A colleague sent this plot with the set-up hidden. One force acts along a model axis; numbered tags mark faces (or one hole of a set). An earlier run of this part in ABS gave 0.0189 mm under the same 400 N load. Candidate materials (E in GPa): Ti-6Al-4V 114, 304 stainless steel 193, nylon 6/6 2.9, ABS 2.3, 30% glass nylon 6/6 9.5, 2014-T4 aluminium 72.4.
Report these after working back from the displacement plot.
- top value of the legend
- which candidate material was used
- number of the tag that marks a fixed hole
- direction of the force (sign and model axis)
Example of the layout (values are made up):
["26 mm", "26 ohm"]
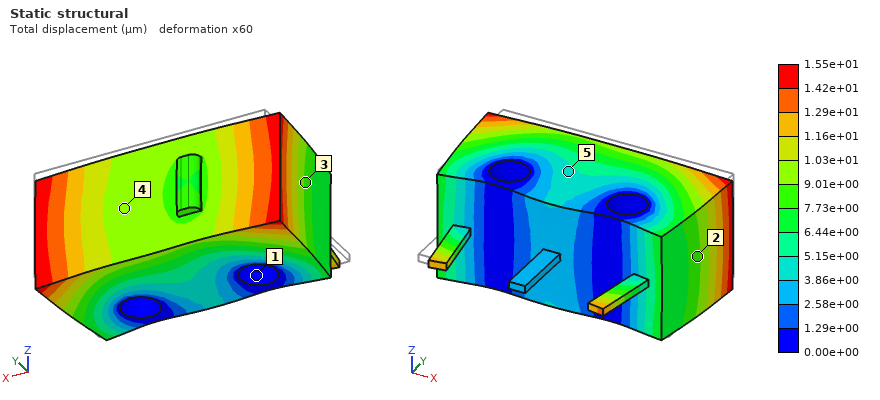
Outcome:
["1.55e+01 µm", "nylon 6/6", "1", "-Y"]
